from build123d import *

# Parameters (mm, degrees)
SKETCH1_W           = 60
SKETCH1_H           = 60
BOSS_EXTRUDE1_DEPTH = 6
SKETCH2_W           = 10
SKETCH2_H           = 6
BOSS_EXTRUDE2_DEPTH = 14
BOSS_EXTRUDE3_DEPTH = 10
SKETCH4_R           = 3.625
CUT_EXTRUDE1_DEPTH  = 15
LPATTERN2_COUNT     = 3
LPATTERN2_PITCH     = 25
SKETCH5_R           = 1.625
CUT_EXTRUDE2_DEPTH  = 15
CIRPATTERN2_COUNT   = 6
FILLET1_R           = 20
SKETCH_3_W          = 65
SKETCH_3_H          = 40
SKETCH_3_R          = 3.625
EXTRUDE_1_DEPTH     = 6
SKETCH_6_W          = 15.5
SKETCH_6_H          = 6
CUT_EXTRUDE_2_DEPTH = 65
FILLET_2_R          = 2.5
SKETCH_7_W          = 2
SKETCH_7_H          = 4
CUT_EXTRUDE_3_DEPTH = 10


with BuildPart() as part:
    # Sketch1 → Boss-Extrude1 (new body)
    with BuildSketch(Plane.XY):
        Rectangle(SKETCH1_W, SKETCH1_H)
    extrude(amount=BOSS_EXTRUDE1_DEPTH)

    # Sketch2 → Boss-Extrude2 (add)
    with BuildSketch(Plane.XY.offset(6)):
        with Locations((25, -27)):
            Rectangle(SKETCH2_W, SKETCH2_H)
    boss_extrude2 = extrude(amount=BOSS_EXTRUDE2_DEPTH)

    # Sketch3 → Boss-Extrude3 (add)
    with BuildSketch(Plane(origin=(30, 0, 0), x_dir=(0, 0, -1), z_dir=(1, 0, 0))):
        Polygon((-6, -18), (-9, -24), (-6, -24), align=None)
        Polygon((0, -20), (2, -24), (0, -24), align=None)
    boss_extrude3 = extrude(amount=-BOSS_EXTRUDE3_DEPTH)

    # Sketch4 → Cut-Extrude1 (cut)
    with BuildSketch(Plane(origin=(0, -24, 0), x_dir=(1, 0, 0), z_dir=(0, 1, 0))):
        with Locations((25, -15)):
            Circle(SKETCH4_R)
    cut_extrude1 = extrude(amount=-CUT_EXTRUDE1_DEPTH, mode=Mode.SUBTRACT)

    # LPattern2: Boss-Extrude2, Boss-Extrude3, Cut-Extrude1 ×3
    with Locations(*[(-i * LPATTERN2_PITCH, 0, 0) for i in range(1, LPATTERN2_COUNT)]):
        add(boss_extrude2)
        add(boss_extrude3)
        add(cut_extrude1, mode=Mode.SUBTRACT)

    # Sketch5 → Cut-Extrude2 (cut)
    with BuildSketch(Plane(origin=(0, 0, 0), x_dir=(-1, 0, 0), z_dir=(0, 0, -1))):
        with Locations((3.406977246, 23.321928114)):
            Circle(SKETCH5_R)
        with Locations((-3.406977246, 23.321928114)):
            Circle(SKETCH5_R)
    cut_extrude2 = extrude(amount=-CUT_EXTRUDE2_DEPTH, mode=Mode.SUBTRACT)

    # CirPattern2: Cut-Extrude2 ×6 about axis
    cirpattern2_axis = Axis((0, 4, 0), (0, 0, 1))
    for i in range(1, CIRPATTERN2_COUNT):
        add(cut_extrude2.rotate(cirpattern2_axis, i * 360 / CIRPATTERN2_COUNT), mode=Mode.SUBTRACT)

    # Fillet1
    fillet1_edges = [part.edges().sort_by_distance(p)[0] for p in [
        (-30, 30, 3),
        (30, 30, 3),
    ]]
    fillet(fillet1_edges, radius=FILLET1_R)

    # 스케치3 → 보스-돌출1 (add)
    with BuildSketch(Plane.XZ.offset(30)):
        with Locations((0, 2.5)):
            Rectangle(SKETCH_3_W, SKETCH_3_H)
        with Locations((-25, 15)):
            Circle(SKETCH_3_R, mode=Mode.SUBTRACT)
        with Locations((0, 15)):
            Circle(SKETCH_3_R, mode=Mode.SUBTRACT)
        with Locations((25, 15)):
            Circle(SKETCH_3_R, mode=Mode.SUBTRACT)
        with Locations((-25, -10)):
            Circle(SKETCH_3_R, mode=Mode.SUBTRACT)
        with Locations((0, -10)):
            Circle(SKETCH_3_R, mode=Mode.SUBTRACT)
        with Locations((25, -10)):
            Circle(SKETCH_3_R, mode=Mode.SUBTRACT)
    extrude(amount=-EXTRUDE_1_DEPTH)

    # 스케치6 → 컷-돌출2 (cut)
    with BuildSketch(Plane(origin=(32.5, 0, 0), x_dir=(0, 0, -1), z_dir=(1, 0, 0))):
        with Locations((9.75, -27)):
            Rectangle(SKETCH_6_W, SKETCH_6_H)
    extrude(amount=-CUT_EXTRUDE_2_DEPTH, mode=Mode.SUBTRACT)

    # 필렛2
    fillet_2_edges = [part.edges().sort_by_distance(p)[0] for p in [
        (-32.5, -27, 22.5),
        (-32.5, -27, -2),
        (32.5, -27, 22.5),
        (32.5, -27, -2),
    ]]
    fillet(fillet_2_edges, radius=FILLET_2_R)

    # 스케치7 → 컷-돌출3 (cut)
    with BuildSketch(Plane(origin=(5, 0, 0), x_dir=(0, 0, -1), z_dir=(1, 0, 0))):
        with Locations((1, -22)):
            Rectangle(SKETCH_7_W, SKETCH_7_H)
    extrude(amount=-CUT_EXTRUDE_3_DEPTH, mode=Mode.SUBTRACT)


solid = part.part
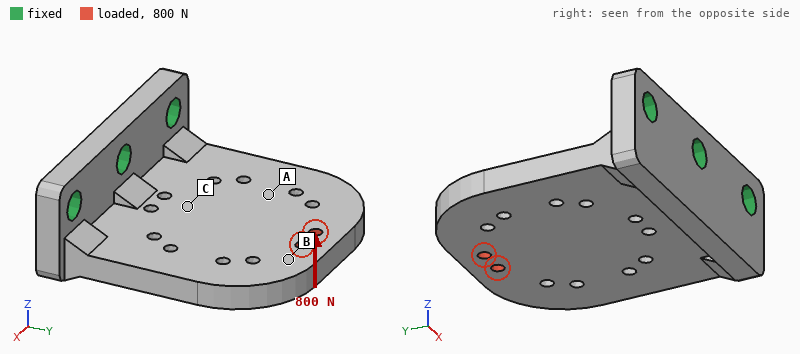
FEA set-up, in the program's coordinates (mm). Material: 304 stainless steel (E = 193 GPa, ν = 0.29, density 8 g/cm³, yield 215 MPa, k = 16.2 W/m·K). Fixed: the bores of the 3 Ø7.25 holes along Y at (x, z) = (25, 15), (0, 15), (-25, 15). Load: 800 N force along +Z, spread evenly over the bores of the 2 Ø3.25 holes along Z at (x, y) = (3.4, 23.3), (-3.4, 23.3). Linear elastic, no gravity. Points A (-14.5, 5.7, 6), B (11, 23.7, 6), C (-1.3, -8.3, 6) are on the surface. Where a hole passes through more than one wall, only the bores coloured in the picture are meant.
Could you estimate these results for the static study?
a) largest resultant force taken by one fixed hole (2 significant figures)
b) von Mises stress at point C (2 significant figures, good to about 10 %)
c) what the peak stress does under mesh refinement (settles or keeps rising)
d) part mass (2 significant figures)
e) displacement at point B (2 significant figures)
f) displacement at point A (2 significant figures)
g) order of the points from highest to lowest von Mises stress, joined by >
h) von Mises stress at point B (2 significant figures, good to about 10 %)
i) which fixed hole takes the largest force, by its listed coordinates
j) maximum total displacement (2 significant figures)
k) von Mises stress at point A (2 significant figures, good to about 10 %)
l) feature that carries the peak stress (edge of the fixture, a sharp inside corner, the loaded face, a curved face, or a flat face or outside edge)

630 N
65 MPa
keeps rising
220 g
0.21 mm
0.11 mm
C > A > B
18 MPa
(0, 15)
0.25 mm
42 MPa
a sharp inside corner
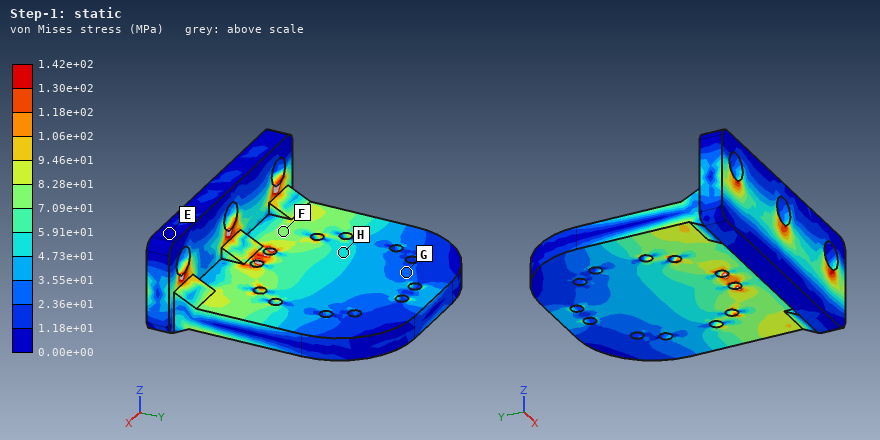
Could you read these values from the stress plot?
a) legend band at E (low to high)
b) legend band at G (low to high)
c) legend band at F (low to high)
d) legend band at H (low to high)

0.00e+00 to 1.18e+01 MPa
2.36e+01 to 3.55e+01 MPa
7.09e+01 to 8.28e+01 MPa
4.73e+01 to 5.91e+01 MPa
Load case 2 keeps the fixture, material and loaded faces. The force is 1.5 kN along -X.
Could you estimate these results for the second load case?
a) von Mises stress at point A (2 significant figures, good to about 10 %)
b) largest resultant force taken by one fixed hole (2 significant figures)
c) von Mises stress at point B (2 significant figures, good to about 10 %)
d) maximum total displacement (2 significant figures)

12 MPa
1.5 kN
8.8 MPa
22 µm
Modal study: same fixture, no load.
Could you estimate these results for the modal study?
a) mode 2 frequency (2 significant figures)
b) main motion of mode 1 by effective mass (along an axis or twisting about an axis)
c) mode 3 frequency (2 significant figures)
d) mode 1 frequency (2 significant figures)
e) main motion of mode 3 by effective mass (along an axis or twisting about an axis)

3700 Hz
along Z
6100 Hz
1400 Hz
along X
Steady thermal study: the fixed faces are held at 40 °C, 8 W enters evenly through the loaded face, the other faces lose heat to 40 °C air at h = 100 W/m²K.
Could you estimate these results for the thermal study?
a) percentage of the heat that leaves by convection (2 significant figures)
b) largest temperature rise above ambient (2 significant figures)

92 %
43 K
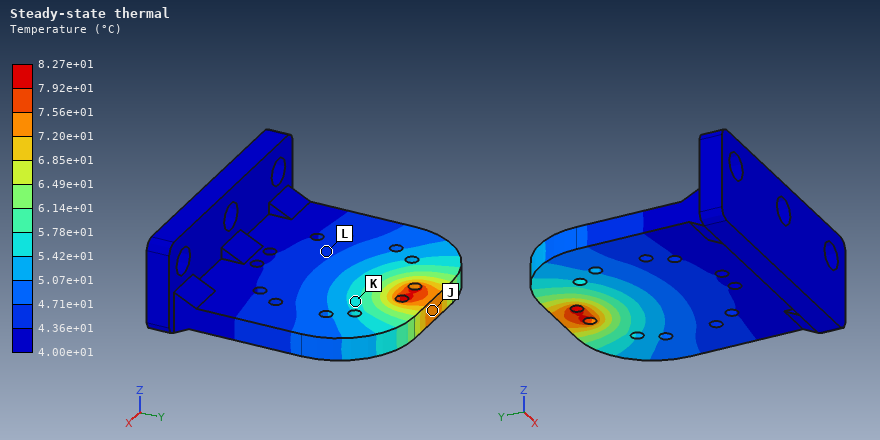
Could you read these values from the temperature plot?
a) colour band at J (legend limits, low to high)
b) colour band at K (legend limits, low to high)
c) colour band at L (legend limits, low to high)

7.20e+01 to 7.56e+01 °C
5.42e+01 to 5.78e+01 °C
4.36e+01 to 4.71e+01 °C
